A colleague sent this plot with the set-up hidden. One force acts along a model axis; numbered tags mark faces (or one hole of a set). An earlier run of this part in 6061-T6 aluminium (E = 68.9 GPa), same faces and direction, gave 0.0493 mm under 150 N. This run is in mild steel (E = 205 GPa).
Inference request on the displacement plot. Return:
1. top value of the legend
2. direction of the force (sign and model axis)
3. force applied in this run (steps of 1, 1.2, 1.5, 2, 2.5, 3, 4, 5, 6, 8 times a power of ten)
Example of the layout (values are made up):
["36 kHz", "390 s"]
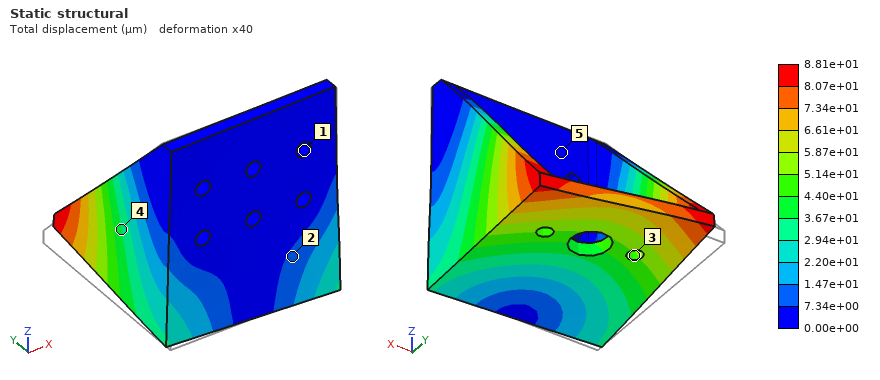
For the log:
["8.81e+01 µm", "+X", "800 N"]
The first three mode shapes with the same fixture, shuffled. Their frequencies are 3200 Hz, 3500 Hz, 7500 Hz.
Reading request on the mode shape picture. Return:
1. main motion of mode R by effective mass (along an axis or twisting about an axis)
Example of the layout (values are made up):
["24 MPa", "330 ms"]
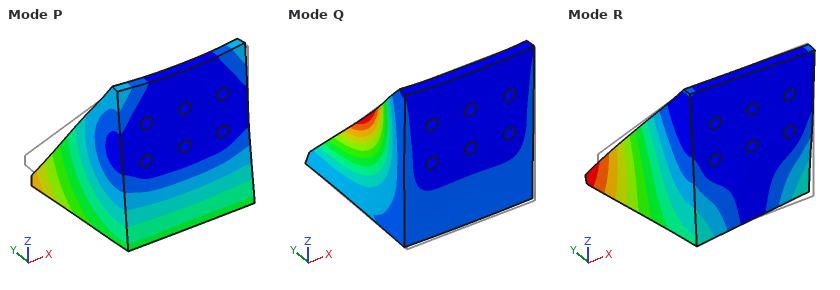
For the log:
["along X"]
